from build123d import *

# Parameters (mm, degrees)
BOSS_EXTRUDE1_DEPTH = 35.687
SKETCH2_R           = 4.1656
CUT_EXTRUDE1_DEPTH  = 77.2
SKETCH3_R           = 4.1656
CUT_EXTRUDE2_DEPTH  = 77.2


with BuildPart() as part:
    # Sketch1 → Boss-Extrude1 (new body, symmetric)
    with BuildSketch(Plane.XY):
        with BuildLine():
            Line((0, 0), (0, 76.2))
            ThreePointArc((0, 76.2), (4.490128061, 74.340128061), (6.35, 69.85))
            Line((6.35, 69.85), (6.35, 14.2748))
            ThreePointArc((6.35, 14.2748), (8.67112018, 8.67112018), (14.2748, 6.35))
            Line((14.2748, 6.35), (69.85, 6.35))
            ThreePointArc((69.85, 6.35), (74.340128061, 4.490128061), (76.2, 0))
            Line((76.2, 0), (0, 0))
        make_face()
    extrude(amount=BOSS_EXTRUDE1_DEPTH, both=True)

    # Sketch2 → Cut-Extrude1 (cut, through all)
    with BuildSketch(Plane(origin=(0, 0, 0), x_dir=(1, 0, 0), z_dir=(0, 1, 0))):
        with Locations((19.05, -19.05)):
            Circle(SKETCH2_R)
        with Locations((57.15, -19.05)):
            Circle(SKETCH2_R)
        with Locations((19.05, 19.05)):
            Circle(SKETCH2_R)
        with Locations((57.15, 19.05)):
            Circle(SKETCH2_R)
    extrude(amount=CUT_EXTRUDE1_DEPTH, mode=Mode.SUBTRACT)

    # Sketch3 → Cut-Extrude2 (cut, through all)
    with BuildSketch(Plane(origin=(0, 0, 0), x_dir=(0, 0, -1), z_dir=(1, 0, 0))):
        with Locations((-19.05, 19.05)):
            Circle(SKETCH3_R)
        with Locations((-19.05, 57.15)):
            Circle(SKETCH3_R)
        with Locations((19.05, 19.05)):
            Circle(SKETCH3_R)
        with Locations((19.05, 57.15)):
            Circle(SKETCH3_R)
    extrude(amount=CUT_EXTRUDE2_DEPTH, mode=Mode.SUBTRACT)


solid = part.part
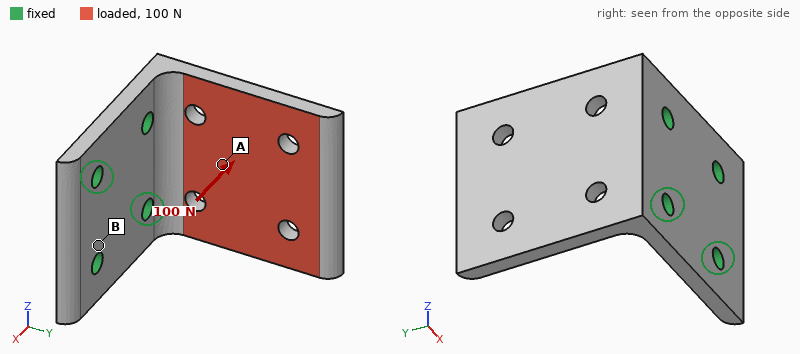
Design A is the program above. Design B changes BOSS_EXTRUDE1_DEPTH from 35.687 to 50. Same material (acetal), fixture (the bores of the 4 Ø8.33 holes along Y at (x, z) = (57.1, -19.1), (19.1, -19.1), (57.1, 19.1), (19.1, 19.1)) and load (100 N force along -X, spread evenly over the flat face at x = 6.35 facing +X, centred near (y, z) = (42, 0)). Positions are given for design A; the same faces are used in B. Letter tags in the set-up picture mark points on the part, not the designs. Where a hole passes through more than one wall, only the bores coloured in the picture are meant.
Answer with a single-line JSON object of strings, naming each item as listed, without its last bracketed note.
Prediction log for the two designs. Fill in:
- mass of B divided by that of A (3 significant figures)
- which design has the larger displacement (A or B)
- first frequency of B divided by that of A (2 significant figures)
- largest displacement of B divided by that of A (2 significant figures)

{"mass of B divided by that of A": "1.42", "which design has the larger displacement": "A", "first frequency of B divided by that of A": "0.98", "largest displacement of B divided by that of A": "0.74"}
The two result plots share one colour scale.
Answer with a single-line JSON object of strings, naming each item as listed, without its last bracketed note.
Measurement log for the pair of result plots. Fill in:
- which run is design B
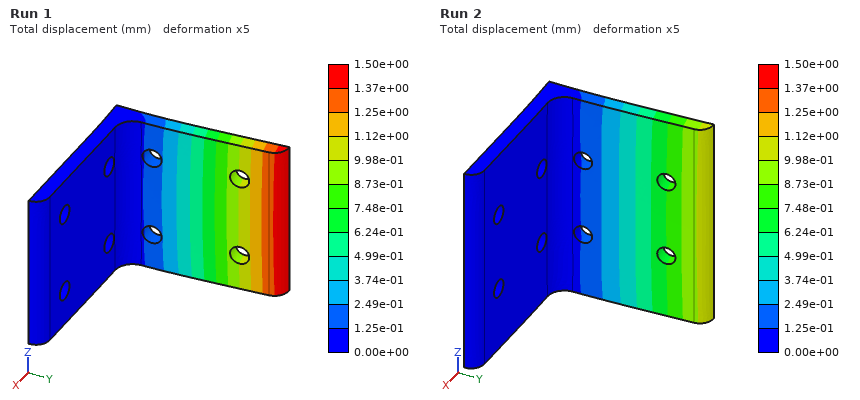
{"which run is design B": "Run 2"}
